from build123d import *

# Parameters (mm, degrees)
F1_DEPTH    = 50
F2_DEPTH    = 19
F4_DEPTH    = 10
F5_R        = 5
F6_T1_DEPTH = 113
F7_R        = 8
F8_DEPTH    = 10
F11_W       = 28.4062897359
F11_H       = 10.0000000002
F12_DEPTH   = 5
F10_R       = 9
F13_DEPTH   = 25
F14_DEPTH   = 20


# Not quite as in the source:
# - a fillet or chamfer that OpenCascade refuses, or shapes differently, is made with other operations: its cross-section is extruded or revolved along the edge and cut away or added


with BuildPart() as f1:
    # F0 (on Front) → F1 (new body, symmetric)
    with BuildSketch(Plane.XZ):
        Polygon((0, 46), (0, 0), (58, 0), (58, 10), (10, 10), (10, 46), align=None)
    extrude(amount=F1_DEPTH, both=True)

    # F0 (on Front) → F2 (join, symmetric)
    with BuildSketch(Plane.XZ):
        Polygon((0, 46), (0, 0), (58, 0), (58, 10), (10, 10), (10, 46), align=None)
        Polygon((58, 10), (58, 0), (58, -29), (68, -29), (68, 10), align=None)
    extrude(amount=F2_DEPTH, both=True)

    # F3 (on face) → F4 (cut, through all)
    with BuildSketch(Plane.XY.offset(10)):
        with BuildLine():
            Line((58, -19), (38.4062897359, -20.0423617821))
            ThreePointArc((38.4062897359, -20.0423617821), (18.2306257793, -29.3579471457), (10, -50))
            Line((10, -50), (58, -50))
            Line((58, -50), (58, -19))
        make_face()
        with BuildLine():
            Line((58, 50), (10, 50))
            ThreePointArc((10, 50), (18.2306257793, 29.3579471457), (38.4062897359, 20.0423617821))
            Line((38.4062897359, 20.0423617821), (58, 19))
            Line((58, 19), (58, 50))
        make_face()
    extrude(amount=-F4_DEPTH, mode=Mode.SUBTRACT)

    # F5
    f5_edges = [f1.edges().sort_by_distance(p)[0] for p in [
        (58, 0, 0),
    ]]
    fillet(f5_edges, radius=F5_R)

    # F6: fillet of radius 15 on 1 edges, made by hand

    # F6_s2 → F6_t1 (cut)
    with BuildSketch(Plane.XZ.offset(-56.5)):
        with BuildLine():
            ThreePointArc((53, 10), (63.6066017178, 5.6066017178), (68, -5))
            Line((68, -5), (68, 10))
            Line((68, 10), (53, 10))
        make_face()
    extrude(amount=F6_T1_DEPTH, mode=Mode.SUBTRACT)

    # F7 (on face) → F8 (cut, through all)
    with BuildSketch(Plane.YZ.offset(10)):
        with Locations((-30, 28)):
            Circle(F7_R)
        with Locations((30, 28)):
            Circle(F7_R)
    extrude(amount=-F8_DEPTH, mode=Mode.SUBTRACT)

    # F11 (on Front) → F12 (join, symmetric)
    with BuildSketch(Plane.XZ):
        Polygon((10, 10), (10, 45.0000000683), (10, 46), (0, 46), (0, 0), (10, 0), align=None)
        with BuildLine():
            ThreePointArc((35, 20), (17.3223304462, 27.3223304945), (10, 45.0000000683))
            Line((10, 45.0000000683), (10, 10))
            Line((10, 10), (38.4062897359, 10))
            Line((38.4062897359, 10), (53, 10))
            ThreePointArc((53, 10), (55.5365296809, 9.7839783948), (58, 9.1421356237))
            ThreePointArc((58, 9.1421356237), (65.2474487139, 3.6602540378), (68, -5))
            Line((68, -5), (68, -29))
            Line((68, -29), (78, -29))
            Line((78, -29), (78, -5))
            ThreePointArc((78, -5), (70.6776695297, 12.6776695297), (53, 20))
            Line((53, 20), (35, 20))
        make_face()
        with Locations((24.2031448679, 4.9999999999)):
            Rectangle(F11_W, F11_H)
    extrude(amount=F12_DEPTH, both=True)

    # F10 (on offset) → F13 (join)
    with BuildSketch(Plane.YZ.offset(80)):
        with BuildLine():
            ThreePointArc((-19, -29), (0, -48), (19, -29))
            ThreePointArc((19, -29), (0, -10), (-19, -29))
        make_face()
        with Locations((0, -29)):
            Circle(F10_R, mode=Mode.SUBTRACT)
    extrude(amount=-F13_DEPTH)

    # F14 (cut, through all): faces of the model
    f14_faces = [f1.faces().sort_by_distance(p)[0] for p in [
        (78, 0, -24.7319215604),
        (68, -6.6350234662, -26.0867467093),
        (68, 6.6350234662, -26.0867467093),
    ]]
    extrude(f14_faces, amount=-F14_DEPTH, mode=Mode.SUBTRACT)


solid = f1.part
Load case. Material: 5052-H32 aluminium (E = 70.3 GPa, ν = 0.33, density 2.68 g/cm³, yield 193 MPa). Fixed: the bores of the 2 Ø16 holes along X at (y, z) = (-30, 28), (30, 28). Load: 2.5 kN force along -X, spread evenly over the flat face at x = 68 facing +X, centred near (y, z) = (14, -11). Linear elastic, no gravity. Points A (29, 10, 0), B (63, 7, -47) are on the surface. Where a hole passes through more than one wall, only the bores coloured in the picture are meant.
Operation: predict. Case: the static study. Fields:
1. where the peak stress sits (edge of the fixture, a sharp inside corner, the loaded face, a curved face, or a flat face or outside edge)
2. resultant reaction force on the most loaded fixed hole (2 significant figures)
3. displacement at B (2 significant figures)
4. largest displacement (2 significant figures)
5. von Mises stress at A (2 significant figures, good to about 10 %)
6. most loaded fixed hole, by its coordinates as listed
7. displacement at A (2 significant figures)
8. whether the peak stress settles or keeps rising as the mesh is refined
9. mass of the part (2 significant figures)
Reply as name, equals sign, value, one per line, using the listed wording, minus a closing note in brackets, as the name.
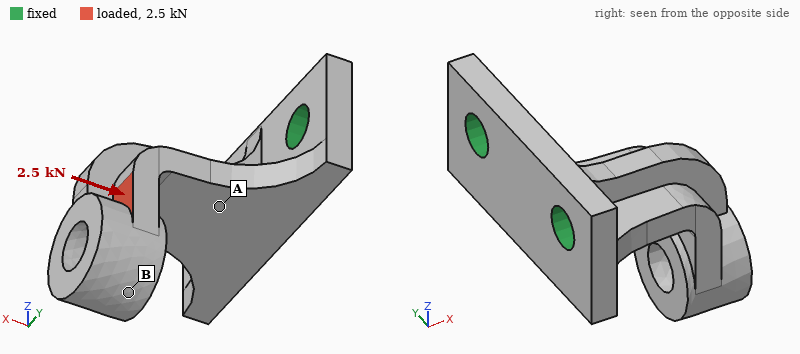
where the peak stress sits = edge of the fixture
resultant reaction force on the most loaded fixed hole = 1.9 kN
displacement at B = 0.29 mm
largest displacement = 0.32 mm
von Mises stress at A = 27 MPa
most loaded fixed hole, by its coordinates as listed = (30, 28)
displacement at A = 0.052 mm
whether the peak stress settles or keeps rising as the mesh is refined = keeps rising
mass of the part = 280 g
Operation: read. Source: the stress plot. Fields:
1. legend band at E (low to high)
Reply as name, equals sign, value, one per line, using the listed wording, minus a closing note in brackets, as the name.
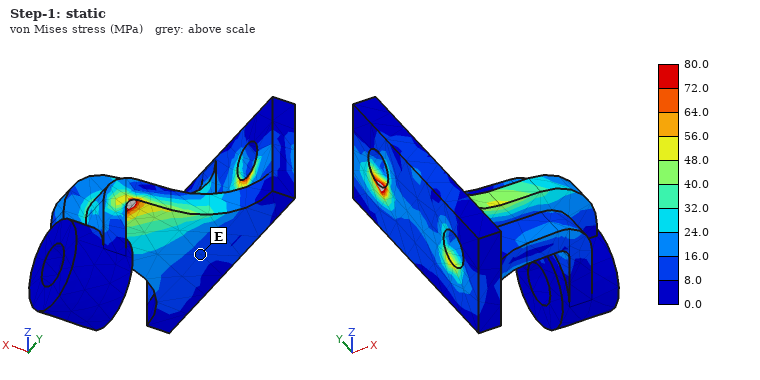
legend band at E = 8.0 to 16.0 MPa
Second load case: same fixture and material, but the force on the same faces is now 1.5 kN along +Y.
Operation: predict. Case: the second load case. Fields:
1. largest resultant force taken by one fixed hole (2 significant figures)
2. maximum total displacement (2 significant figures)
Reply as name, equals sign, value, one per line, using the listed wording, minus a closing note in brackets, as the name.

largest resultant force taken by one fixed hole = 1.9 kN
maximum total displacement = 0.15 mm
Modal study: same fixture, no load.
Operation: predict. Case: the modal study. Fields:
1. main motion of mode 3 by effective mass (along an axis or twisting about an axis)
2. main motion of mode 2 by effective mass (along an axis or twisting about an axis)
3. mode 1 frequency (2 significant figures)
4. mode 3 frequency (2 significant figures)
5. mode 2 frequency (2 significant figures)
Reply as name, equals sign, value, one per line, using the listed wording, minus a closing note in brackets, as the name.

main motion of mode 3 by effective mass = along Z
main motion of mode 2 by effective mass = along Y
mode 1 frequency = 1200 Hz
mode 3 frequency = 3500 Hz
mode 2 frequency = 1600 Hz
